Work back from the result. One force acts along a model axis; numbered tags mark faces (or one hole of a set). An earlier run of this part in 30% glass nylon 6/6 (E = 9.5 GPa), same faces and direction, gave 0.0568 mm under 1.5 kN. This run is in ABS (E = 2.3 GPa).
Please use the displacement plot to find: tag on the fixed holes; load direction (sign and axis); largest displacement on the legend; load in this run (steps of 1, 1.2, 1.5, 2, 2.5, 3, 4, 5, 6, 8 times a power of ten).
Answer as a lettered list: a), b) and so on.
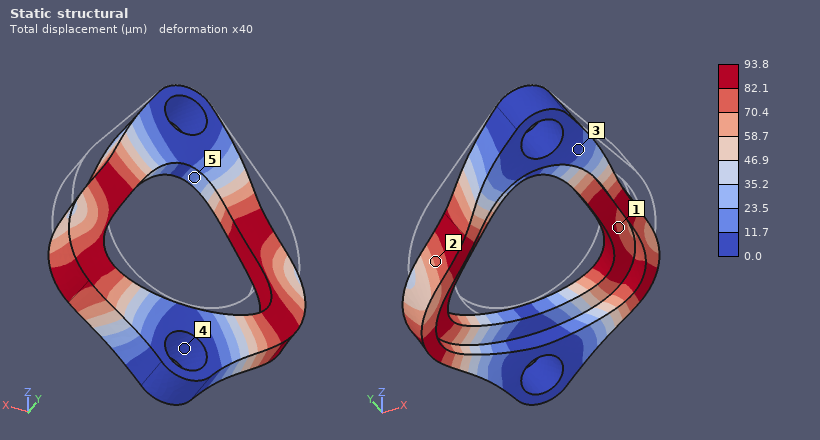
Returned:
a) 4
b) -Z
c) 93.8 µm
d) 600 N
